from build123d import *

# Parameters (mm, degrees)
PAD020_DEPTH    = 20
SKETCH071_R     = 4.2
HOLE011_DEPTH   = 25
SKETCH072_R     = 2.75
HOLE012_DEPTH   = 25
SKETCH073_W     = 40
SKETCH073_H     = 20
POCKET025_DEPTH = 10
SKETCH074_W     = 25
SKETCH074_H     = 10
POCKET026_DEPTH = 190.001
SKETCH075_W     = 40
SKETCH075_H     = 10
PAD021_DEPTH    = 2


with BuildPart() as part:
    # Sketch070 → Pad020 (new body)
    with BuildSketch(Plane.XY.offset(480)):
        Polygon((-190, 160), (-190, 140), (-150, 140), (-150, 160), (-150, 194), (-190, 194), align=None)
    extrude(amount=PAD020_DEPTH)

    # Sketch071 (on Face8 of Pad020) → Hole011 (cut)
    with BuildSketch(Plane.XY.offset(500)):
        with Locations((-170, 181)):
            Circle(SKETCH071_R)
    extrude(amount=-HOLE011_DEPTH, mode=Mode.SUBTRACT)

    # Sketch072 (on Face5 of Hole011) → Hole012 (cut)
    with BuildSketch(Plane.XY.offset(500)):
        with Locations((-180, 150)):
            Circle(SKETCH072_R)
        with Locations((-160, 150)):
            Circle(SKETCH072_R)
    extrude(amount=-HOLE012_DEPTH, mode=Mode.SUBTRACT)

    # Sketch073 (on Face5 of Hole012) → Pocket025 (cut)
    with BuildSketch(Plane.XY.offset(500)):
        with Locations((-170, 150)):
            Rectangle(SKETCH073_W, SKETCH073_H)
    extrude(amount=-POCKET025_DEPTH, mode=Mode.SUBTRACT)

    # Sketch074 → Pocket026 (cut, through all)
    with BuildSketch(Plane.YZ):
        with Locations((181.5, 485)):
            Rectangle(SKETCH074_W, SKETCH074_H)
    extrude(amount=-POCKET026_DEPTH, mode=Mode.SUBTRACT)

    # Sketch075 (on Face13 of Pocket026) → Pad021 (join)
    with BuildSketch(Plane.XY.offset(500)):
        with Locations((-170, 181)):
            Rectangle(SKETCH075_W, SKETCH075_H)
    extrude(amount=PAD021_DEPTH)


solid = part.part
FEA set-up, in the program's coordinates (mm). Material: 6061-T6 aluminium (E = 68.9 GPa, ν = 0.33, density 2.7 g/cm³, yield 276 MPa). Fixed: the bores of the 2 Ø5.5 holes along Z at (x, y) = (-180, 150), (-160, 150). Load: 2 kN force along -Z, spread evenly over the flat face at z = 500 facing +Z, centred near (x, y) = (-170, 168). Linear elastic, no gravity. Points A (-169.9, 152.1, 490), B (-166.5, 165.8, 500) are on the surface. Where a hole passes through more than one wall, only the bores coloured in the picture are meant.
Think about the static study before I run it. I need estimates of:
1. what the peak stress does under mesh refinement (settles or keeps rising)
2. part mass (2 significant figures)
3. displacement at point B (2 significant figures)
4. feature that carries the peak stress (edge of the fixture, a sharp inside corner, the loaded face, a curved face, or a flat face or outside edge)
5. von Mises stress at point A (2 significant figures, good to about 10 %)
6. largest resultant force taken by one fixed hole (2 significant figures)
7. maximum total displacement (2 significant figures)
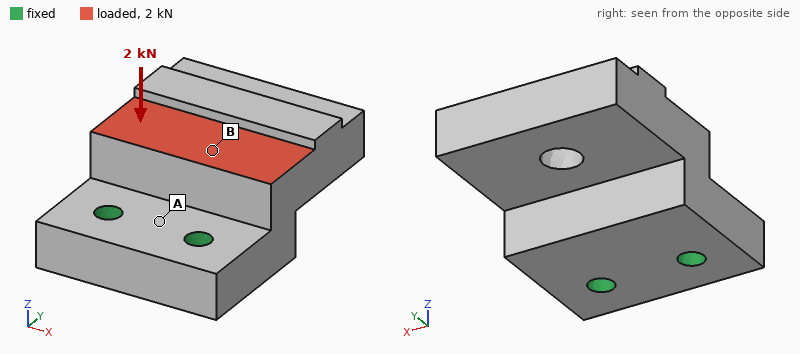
keeps rising
67 g
29 µm
edge of the fixture
22 MPa
1.0 kN
68 µm
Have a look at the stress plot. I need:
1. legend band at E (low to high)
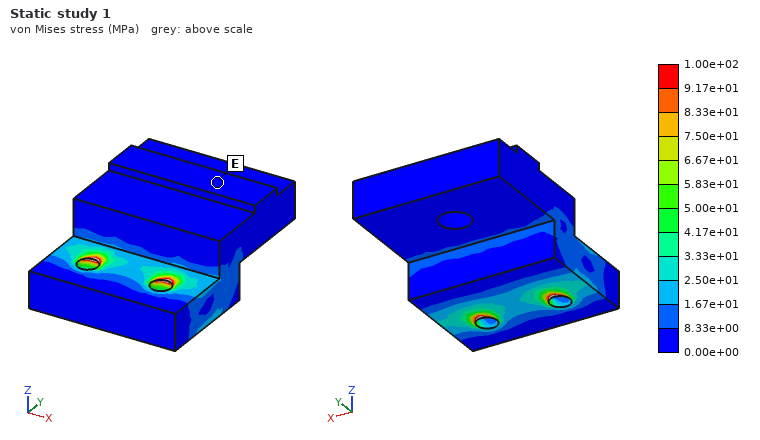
0.00e+00 to 8.33e+00 MPa
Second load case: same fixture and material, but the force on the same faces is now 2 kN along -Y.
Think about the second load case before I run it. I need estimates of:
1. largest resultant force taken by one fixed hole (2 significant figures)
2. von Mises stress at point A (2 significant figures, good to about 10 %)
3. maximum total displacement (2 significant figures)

1.0 kN
25 MPa
94 µm
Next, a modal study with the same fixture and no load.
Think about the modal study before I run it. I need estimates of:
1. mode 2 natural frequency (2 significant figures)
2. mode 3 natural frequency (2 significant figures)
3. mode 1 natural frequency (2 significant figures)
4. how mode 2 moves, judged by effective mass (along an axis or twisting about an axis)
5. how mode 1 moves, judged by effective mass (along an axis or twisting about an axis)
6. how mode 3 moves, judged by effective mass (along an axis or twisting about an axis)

8200 Hz
9100 Hz
3500 Hz
along X
along Z
along X
